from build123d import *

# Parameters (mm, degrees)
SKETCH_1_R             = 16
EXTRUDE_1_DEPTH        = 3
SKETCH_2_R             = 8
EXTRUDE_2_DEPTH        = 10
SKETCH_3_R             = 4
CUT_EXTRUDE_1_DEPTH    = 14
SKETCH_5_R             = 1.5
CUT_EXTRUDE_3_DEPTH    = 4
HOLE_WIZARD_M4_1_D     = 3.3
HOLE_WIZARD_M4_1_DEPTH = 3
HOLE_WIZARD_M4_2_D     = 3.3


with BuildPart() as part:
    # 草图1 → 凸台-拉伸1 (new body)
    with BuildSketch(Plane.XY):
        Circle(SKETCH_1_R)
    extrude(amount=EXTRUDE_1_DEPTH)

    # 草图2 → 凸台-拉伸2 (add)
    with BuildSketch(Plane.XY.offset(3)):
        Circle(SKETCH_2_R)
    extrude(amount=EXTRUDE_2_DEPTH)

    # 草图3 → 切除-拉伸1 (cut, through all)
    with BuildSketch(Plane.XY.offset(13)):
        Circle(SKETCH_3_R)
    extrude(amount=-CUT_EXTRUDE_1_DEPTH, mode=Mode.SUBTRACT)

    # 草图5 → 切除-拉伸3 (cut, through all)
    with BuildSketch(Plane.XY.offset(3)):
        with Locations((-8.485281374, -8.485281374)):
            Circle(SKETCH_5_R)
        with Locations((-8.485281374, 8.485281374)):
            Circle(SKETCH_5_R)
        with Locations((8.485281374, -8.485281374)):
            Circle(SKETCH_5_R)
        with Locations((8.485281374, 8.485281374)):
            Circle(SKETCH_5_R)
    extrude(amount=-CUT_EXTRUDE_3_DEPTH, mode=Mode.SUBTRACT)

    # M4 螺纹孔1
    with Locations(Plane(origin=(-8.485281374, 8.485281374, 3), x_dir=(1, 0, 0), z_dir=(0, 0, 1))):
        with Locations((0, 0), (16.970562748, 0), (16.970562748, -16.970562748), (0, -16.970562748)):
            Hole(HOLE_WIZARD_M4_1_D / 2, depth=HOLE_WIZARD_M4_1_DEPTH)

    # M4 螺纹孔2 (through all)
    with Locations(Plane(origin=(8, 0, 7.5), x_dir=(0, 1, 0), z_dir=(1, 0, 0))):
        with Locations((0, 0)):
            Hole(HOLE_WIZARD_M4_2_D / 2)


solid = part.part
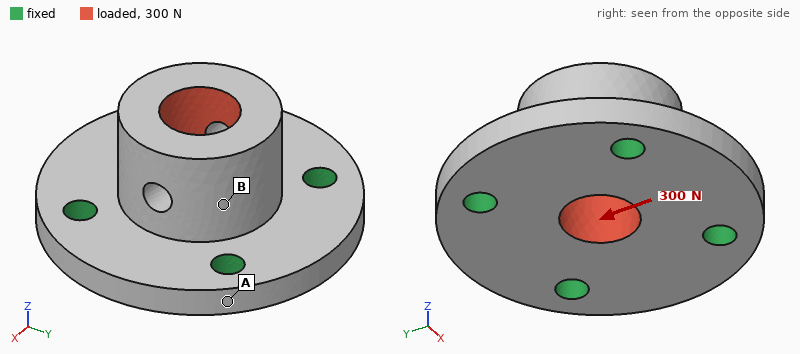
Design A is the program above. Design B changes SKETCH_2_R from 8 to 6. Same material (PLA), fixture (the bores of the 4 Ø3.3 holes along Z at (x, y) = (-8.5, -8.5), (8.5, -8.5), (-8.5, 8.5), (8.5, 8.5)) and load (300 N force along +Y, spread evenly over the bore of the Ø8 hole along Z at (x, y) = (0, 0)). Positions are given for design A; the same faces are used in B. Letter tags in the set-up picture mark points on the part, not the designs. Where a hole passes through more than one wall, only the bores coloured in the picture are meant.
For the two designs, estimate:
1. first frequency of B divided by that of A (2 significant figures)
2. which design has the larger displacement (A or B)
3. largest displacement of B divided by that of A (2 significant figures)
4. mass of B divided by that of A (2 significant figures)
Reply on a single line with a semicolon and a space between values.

0.96; B; 2.7; 0.77
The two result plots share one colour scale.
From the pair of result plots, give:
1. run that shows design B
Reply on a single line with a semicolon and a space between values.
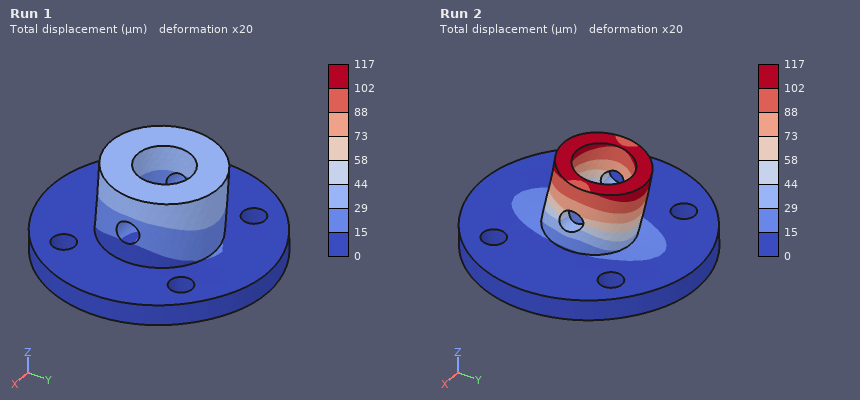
Run 2
